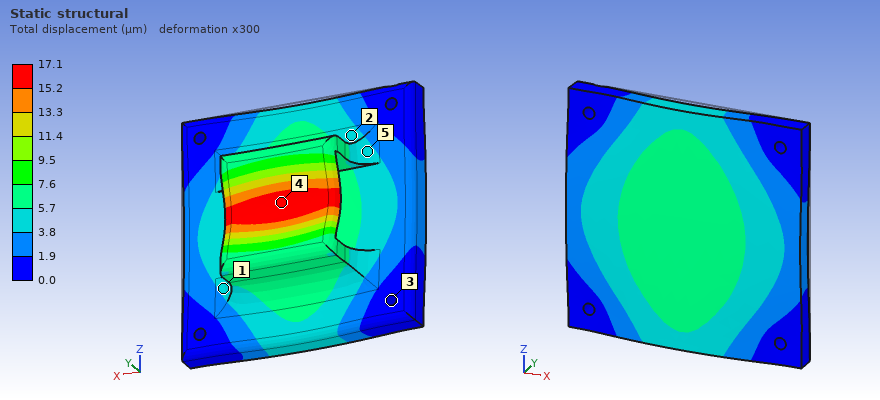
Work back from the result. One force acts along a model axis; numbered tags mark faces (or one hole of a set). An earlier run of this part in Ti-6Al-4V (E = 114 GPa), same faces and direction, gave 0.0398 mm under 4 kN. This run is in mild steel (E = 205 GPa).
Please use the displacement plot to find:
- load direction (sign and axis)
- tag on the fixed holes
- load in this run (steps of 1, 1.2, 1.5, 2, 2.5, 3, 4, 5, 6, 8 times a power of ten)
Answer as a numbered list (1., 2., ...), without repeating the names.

1. -Y
2. 3
3. 3 kN
